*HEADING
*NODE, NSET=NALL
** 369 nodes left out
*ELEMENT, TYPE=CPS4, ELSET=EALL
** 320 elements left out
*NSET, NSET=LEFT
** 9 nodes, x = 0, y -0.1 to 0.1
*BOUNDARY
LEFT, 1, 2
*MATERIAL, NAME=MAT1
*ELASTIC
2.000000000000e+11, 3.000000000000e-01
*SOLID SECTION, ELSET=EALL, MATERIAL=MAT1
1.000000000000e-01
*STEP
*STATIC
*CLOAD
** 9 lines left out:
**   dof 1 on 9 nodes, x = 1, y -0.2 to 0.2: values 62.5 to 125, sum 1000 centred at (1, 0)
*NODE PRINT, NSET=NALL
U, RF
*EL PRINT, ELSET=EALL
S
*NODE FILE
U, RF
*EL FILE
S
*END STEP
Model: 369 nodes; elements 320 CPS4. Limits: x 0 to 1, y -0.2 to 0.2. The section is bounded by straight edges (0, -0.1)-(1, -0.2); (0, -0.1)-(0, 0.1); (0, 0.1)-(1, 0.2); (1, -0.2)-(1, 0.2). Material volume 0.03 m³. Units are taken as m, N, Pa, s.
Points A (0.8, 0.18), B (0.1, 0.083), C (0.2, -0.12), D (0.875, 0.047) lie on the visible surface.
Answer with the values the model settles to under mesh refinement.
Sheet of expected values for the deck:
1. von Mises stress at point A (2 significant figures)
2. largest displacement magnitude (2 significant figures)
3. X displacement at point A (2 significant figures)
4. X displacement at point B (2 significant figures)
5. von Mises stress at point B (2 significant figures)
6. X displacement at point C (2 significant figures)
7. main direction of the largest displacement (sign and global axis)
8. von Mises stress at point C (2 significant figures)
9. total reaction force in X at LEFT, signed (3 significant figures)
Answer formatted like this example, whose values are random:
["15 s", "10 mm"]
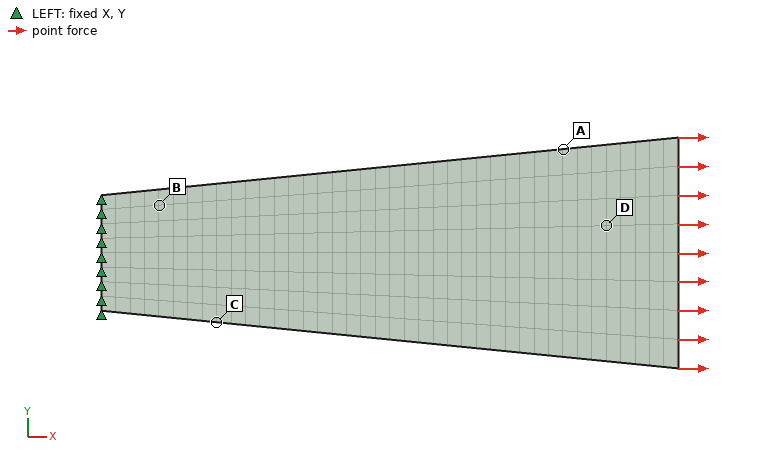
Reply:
["29000 Pa", "2.0e-07 m", "1.5e-07 m", "2.4e-08 m", "45000 Pa", "4.7e-08 m", "+X", "41000 Pa", "-1000 N"]
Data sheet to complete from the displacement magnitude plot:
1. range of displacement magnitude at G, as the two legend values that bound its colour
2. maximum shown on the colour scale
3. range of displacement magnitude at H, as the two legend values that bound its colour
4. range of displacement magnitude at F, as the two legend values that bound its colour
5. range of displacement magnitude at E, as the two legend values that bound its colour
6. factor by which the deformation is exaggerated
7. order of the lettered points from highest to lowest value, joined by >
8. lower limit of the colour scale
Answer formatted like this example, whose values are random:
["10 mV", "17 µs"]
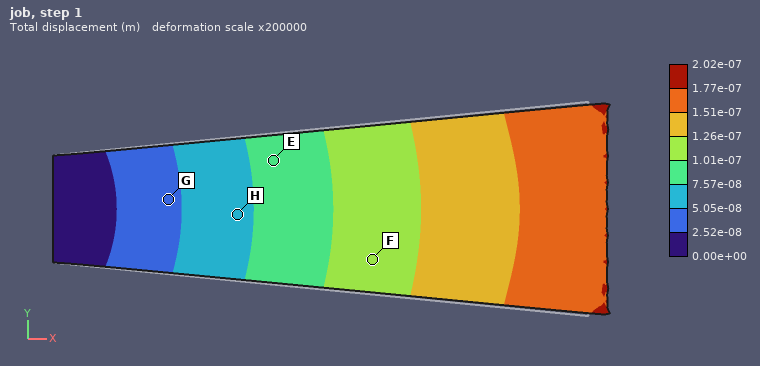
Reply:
["2.52e-08 to 5.05e-08 m", "2.02e-07 m", "5.05e-08 to 7.57e-08 m", "1.01e-07 to 1.26e-07 m", "7.57e-08 to 1.01e-07 m", "200000", "F > E > H > G", "0.00e+00 m"]
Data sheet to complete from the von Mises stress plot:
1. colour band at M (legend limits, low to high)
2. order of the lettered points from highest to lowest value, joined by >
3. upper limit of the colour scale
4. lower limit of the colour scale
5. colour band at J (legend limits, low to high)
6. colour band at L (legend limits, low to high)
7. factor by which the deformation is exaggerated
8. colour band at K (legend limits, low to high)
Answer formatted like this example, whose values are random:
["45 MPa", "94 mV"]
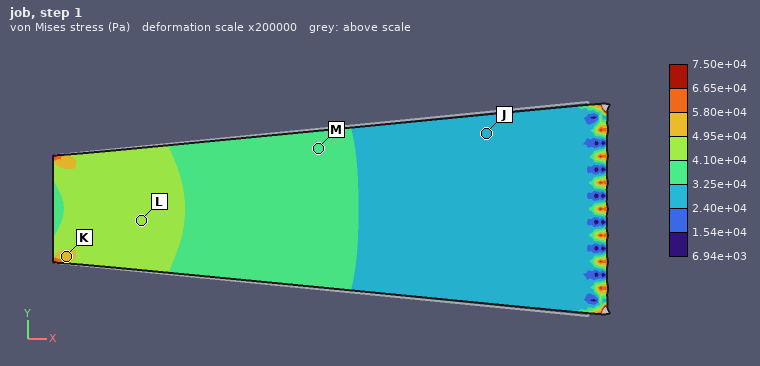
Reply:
["3.25e+04 to 4.10e+04 Pa", "K > L > M > J", "7.50e+04 Pa", "6.94e+03 Pa", "2.40e+04 to 3.25e+04 Pa", "4.10e+04 to 4.95e+04 Pa", "200000", "4.95e+04 to 5.80e+04 Pa"]
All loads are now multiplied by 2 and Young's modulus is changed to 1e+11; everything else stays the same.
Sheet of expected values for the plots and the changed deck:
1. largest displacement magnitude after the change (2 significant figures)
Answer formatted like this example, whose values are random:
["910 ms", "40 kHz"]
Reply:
["8.1e-07 m"]
